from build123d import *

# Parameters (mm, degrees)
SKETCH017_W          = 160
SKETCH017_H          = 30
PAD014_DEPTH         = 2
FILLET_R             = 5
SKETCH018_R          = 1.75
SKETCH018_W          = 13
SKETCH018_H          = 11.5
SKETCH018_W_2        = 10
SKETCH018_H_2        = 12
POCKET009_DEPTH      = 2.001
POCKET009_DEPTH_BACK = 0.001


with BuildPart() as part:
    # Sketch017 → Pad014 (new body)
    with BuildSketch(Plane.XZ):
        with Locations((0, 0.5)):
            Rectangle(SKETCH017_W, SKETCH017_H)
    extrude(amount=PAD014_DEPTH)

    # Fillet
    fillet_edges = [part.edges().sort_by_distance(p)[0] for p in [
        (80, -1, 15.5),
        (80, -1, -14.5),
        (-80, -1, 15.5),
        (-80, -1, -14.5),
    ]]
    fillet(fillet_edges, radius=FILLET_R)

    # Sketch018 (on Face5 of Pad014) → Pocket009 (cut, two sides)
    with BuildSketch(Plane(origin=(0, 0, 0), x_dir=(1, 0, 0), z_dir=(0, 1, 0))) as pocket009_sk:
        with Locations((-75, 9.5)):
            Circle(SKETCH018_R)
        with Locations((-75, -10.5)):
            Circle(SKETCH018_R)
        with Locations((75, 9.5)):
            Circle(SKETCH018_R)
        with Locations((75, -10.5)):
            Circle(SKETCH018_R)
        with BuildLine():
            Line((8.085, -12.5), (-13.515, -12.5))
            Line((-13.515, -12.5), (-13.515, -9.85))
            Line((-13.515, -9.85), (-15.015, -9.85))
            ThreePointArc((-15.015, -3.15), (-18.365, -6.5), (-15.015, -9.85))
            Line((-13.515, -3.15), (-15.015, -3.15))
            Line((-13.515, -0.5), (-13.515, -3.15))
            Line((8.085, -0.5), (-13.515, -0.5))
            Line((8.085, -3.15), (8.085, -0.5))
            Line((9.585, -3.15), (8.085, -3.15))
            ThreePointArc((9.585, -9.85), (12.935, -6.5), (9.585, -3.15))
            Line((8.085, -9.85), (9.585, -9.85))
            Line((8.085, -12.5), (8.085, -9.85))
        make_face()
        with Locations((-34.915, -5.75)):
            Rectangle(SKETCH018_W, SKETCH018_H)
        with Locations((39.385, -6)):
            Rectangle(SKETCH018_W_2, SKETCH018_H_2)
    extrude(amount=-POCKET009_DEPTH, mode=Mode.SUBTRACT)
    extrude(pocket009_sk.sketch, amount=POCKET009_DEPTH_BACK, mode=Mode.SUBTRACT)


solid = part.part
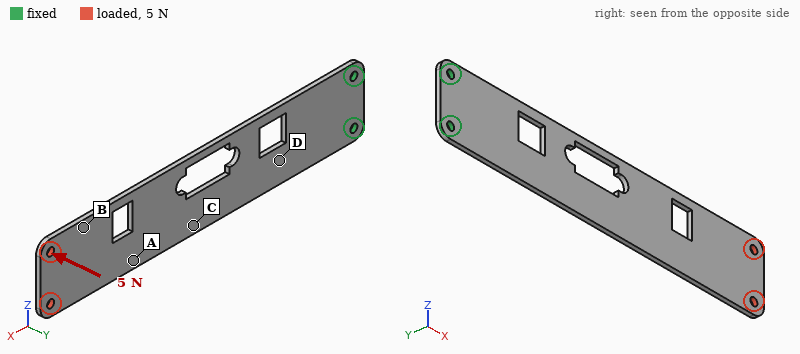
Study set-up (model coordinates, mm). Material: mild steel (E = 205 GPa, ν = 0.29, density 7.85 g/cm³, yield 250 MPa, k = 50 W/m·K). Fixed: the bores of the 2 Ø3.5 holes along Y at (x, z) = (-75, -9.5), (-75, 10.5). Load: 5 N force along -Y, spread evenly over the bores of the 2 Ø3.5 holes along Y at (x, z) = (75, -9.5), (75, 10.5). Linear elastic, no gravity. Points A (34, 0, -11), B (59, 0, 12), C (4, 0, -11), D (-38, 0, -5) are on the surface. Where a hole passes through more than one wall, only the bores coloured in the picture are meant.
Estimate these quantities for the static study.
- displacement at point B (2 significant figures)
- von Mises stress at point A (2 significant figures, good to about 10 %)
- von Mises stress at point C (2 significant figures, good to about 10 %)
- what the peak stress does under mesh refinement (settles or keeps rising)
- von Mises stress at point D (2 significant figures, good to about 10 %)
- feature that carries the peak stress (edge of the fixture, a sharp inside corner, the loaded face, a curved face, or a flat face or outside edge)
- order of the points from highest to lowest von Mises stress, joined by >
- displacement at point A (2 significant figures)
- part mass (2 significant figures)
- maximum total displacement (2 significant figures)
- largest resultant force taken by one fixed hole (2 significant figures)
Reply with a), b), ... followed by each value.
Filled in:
a) 1.4 mm
b) 14 MPa
c) 28 MPa
d) keeps rising
e) 45 MPa
f) edge of the fixture
g) D > C > A > B
h) 1.00 mm
i) 65 g
j) 1.8 mm
k) 2.5 N
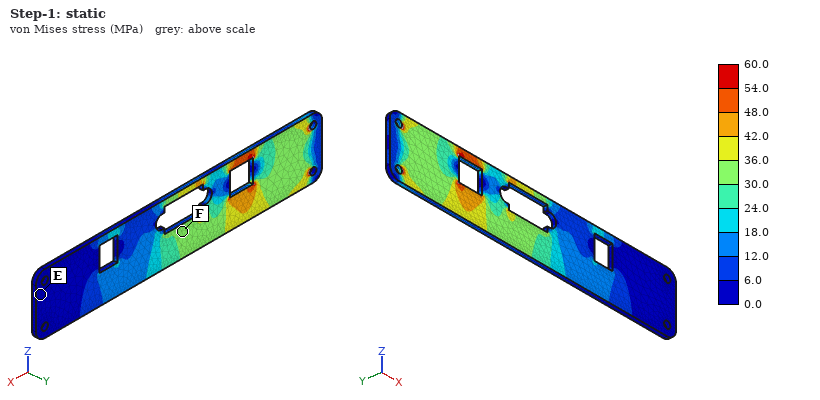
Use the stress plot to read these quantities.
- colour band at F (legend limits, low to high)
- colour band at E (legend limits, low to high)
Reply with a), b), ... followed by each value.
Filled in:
a) 30.0 to 36.0 MPa
b) 0.0 to 6.0 MPa
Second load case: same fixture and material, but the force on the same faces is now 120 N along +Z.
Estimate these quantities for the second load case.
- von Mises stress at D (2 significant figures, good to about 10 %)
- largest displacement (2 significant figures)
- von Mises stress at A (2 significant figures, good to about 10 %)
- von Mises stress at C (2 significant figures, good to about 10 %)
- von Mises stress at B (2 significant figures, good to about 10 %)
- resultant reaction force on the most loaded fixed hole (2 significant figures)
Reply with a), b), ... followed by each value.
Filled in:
a) 14 MPa
b) 0.21 mm
c) 15 MPa
d) 20 MPa
e) 7.4 MPa
f) 840 N
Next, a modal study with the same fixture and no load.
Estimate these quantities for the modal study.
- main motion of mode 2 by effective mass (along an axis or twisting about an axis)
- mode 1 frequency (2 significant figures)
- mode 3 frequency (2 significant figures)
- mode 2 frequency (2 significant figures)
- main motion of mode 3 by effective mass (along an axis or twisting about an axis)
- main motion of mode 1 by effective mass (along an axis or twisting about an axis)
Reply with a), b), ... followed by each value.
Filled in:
a) along Y
b) 66 Hz
c) 650 Hz
d) 420 Hz
e) twisting about X
f) along Y
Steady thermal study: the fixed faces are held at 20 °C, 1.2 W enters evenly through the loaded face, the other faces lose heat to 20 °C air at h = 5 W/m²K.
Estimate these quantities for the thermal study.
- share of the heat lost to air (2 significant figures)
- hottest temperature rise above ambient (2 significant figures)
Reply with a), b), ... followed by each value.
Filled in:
a) 66 %
b) 41 K
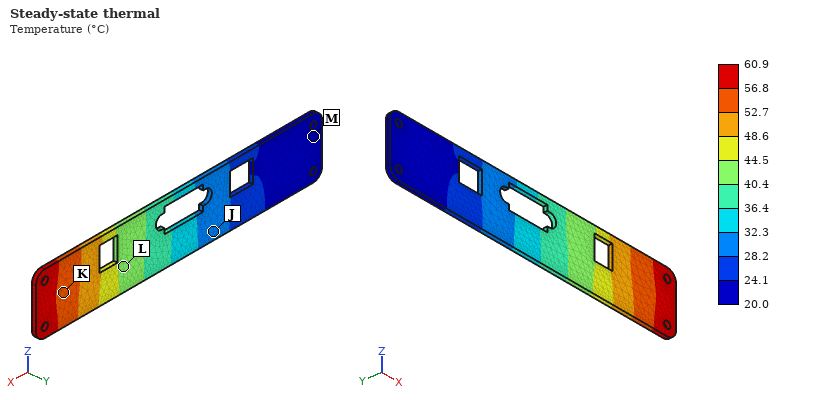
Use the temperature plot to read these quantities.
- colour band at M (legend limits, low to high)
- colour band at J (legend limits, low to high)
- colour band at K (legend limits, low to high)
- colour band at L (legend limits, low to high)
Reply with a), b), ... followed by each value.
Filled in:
a) 20.0 to 24.1 °C
b) 28.2 to 32.3 °C
c) 52.7 to 56.8 °C
d) 40.4 to 44.5 °C
